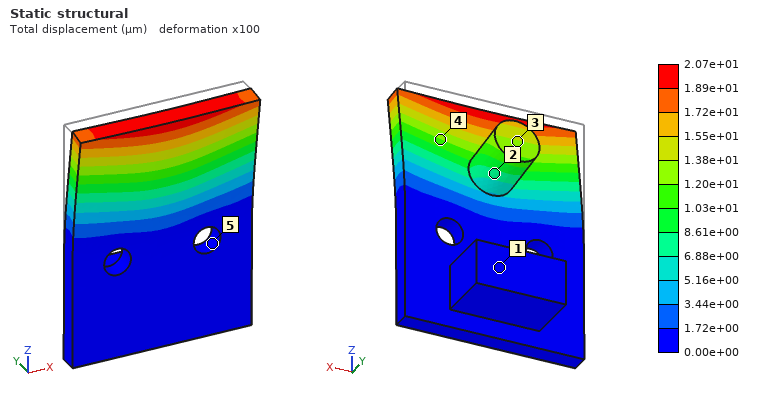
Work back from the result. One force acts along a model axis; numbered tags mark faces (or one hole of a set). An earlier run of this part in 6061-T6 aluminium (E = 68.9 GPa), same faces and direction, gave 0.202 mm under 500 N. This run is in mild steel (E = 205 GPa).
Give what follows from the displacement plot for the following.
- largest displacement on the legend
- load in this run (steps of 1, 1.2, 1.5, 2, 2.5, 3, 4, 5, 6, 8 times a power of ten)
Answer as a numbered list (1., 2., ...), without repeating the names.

1. 2.07e+01 µm
2. 150 N
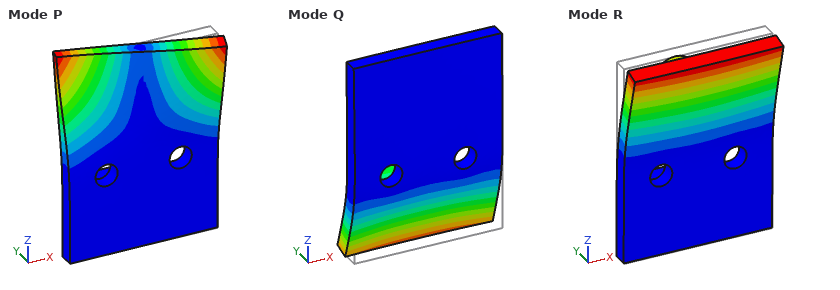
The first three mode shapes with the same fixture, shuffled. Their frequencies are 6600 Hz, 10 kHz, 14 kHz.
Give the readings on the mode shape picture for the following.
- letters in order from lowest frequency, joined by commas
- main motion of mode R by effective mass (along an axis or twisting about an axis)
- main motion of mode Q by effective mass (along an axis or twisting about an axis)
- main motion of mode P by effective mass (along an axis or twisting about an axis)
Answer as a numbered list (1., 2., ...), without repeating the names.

1. R, Q, P
2. along Y
3. along Y
4. twisting about Z
